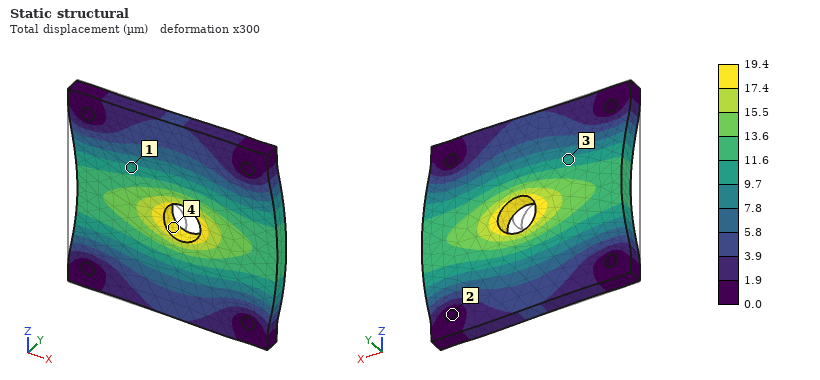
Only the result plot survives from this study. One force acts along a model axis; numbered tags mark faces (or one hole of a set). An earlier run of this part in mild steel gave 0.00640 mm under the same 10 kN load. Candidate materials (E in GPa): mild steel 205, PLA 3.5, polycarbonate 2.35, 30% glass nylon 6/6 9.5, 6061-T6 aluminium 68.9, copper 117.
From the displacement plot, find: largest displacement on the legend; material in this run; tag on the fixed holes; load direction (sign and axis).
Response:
19.4 µm
6061-T6 aluminium
2
+X
